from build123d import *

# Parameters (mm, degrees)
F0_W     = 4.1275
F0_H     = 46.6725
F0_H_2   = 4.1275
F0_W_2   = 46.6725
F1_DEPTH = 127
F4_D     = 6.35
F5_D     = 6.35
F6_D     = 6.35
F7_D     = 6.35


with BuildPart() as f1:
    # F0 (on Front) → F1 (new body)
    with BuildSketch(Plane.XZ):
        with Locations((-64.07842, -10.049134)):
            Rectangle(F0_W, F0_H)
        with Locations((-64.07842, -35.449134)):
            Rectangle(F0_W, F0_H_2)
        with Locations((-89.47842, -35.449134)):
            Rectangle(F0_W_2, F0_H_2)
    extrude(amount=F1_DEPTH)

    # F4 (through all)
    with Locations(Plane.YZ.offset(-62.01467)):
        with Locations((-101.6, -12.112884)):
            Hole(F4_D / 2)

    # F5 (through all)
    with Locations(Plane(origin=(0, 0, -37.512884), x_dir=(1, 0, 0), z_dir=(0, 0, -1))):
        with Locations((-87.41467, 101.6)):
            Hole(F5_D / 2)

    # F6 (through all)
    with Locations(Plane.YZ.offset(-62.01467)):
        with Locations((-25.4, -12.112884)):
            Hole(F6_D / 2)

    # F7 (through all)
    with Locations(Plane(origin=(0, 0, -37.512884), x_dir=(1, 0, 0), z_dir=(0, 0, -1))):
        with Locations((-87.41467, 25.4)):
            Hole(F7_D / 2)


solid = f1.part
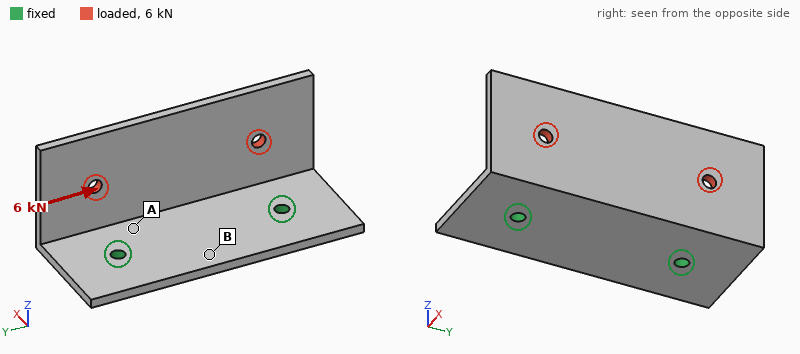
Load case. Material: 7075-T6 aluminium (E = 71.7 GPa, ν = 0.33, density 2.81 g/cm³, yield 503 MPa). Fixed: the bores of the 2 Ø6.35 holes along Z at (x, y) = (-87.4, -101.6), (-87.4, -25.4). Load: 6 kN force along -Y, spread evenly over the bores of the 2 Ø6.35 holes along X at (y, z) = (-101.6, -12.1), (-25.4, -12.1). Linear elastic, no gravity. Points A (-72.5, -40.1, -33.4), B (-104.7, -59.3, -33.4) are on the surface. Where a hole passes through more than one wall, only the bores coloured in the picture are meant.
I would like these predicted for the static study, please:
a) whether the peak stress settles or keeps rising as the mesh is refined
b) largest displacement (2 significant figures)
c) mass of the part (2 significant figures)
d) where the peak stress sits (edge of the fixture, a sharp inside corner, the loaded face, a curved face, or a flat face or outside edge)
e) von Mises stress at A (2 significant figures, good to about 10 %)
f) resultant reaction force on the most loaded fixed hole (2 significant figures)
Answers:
keeps rising
0.75 mm
140 g
edge of the fixture
110 MPa
3.9 kN
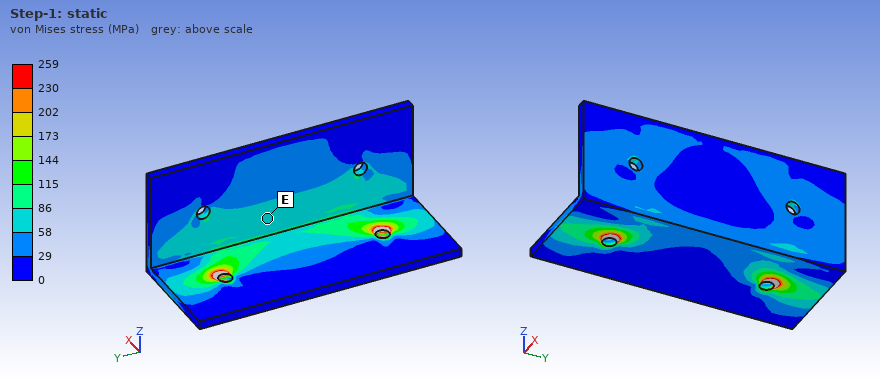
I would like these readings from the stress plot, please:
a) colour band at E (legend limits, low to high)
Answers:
58 to 86 MPa
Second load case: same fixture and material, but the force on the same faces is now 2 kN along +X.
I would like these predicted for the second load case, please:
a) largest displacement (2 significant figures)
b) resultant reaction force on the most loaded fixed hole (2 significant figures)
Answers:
1.5 mm
1.0 kN
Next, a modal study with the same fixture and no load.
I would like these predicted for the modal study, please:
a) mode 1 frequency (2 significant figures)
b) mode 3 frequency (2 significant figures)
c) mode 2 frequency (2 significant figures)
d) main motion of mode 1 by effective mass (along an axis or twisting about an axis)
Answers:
770 Hz
2300 Hz
1300 Hz
along X
